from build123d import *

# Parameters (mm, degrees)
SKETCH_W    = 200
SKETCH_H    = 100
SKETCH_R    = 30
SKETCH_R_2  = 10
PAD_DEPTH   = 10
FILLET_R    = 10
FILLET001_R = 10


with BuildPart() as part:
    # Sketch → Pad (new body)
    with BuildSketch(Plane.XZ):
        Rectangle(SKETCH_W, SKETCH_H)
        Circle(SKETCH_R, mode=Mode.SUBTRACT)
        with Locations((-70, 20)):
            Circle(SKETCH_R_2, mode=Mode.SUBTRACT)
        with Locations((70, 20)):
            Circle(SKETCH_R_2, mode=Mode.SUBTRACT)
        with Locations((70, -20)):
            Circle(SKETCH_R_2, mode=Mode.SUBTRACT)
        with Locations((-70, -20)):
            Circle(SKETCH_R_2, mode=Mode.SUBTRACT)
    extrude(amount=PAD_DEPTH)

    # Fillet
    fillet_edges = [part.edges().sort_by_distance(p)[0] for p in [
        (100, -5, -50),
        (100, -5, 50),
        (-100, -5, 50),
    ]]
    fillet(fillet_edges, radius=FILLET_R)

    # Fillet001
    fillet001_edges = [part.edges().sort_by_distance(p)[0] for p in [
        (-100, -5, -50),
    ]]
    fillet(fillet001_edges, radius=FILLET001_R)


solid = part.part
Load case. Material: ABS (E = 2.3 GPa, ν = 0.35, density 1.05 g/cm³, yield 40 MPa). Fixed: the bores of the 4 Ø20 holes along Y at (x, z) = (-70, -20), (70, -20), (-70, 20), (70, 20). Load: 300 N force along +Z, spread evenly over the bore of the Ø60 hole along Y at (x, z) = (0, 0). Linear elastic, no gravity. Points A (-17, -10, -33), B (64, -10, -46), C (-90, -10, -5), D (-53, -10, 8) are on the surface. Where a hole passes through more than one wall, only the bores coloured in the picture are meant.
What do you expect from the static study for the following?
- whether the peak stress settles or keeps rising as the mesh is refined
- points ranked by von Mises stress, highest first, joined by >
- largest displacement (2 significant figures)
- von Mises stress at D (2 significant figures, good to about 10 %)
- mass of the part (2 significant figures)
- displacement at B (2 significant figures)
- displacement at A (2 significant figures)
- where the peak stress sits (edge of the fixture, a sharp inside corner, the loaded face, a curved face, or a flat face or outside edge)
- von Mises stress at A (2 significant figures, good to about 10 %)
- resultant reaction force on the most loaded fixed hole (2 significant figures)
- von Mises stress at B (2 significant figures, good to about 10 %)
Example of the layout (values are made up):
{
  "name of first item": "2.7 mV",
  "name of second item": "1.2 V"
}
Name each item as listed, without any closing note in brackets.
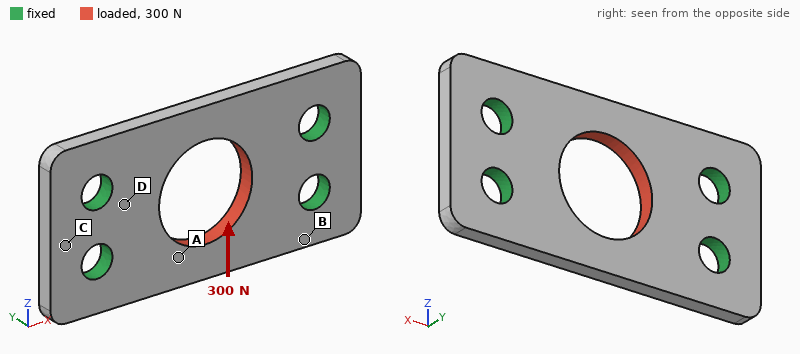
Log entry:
{
  "whether the peak stress settles or keeps rising as the mesh is refined": "keeps rising",
  "points ranked by von Mises stress, highest first, joined by >": "D > A > B > C",
  "largest displacement": "17 µm",
  "von Mises stress at D": "0.43 MPa",
  "mass of the part": "170 g",
  "displacement at B": "2.9 µm",
  "displacement at A": "13 µm",
  "where the peak stress sits": "edge of the fixture",
  "von Mises stress at A": "0.28 MPa",
  "resultant reaction force on the most loaded fixed hole": "88 N",
  "von Mises stress at B": "0.13 MPa"
}
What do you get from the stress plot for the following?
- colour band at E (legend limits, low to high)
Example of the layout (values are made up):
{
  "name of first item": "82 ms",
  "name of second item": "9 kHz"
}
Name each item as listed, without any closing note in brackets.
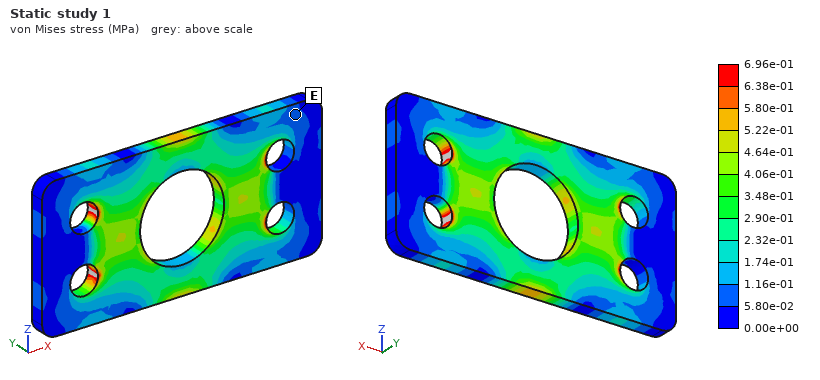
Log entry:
{
  "colour band at E": "5.80e-02 to 1.16e-01 MPa"
}
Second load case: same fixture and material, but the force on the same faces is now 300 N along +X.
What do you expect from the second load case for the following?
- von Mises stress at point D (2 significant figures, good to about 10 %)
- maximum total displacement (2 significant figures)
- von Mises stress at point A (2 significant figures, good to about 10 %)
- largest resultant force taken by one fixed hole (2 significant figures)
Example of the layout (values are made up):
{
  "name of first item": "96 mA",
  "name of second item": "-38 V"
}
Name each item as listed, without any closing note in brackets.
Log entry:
{
  "von Mises stress at point D": "0.15 MPa",
  "maximum total displacement": "5.2 µm",
  "von Mises stress at point A": "0.17 MPa",
  "largest resultant force taken by one fixed hole": "76 N"
}
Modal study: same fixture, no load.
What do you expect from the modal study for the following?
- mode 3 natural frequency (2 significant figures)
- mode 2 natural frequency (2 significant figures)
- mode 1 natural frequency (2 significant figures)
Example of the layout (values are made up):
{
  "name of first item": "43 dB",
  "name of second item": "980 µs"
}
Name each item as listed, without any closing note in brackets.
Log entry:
{
  "mode 3 natural frequency": "2200 Hz",
  "mode 2 natural frequency": "1000 Hz",
  "mode 1 natural frequency": "1000 Hz"
}
